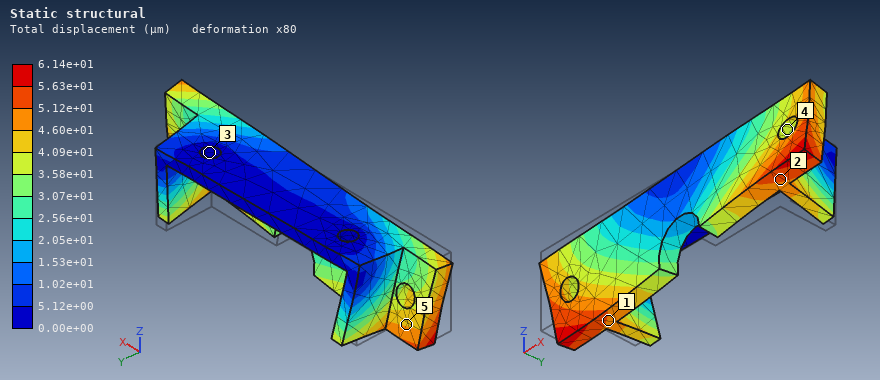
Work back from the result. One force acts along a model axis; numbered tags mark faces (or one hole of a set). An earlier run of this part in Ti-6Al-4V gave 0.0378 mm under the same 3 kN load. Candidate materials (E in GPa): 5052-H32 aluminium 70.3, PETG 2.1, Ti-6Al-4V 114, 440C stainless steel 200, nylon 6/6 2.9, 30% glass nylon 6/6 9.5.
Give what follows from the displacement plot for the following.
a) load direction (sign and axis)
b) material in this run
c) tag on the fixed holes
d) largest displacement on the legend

+X
5052-H32 aluminium
3
6.14e+01 µm
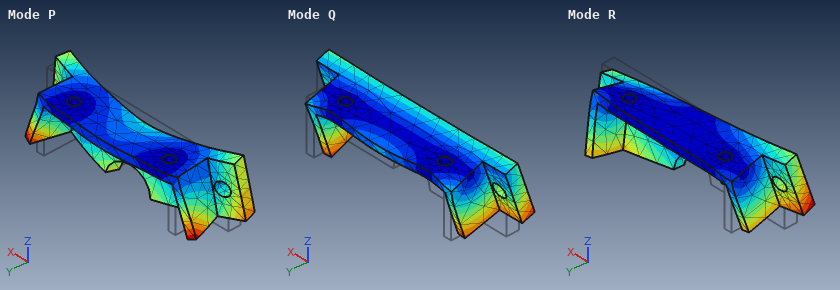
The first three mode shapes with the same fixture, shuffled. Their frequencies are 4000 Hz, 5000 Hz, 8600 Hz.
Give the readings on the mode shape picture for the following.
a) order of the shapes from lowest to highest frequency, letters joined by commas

Q, R, P
